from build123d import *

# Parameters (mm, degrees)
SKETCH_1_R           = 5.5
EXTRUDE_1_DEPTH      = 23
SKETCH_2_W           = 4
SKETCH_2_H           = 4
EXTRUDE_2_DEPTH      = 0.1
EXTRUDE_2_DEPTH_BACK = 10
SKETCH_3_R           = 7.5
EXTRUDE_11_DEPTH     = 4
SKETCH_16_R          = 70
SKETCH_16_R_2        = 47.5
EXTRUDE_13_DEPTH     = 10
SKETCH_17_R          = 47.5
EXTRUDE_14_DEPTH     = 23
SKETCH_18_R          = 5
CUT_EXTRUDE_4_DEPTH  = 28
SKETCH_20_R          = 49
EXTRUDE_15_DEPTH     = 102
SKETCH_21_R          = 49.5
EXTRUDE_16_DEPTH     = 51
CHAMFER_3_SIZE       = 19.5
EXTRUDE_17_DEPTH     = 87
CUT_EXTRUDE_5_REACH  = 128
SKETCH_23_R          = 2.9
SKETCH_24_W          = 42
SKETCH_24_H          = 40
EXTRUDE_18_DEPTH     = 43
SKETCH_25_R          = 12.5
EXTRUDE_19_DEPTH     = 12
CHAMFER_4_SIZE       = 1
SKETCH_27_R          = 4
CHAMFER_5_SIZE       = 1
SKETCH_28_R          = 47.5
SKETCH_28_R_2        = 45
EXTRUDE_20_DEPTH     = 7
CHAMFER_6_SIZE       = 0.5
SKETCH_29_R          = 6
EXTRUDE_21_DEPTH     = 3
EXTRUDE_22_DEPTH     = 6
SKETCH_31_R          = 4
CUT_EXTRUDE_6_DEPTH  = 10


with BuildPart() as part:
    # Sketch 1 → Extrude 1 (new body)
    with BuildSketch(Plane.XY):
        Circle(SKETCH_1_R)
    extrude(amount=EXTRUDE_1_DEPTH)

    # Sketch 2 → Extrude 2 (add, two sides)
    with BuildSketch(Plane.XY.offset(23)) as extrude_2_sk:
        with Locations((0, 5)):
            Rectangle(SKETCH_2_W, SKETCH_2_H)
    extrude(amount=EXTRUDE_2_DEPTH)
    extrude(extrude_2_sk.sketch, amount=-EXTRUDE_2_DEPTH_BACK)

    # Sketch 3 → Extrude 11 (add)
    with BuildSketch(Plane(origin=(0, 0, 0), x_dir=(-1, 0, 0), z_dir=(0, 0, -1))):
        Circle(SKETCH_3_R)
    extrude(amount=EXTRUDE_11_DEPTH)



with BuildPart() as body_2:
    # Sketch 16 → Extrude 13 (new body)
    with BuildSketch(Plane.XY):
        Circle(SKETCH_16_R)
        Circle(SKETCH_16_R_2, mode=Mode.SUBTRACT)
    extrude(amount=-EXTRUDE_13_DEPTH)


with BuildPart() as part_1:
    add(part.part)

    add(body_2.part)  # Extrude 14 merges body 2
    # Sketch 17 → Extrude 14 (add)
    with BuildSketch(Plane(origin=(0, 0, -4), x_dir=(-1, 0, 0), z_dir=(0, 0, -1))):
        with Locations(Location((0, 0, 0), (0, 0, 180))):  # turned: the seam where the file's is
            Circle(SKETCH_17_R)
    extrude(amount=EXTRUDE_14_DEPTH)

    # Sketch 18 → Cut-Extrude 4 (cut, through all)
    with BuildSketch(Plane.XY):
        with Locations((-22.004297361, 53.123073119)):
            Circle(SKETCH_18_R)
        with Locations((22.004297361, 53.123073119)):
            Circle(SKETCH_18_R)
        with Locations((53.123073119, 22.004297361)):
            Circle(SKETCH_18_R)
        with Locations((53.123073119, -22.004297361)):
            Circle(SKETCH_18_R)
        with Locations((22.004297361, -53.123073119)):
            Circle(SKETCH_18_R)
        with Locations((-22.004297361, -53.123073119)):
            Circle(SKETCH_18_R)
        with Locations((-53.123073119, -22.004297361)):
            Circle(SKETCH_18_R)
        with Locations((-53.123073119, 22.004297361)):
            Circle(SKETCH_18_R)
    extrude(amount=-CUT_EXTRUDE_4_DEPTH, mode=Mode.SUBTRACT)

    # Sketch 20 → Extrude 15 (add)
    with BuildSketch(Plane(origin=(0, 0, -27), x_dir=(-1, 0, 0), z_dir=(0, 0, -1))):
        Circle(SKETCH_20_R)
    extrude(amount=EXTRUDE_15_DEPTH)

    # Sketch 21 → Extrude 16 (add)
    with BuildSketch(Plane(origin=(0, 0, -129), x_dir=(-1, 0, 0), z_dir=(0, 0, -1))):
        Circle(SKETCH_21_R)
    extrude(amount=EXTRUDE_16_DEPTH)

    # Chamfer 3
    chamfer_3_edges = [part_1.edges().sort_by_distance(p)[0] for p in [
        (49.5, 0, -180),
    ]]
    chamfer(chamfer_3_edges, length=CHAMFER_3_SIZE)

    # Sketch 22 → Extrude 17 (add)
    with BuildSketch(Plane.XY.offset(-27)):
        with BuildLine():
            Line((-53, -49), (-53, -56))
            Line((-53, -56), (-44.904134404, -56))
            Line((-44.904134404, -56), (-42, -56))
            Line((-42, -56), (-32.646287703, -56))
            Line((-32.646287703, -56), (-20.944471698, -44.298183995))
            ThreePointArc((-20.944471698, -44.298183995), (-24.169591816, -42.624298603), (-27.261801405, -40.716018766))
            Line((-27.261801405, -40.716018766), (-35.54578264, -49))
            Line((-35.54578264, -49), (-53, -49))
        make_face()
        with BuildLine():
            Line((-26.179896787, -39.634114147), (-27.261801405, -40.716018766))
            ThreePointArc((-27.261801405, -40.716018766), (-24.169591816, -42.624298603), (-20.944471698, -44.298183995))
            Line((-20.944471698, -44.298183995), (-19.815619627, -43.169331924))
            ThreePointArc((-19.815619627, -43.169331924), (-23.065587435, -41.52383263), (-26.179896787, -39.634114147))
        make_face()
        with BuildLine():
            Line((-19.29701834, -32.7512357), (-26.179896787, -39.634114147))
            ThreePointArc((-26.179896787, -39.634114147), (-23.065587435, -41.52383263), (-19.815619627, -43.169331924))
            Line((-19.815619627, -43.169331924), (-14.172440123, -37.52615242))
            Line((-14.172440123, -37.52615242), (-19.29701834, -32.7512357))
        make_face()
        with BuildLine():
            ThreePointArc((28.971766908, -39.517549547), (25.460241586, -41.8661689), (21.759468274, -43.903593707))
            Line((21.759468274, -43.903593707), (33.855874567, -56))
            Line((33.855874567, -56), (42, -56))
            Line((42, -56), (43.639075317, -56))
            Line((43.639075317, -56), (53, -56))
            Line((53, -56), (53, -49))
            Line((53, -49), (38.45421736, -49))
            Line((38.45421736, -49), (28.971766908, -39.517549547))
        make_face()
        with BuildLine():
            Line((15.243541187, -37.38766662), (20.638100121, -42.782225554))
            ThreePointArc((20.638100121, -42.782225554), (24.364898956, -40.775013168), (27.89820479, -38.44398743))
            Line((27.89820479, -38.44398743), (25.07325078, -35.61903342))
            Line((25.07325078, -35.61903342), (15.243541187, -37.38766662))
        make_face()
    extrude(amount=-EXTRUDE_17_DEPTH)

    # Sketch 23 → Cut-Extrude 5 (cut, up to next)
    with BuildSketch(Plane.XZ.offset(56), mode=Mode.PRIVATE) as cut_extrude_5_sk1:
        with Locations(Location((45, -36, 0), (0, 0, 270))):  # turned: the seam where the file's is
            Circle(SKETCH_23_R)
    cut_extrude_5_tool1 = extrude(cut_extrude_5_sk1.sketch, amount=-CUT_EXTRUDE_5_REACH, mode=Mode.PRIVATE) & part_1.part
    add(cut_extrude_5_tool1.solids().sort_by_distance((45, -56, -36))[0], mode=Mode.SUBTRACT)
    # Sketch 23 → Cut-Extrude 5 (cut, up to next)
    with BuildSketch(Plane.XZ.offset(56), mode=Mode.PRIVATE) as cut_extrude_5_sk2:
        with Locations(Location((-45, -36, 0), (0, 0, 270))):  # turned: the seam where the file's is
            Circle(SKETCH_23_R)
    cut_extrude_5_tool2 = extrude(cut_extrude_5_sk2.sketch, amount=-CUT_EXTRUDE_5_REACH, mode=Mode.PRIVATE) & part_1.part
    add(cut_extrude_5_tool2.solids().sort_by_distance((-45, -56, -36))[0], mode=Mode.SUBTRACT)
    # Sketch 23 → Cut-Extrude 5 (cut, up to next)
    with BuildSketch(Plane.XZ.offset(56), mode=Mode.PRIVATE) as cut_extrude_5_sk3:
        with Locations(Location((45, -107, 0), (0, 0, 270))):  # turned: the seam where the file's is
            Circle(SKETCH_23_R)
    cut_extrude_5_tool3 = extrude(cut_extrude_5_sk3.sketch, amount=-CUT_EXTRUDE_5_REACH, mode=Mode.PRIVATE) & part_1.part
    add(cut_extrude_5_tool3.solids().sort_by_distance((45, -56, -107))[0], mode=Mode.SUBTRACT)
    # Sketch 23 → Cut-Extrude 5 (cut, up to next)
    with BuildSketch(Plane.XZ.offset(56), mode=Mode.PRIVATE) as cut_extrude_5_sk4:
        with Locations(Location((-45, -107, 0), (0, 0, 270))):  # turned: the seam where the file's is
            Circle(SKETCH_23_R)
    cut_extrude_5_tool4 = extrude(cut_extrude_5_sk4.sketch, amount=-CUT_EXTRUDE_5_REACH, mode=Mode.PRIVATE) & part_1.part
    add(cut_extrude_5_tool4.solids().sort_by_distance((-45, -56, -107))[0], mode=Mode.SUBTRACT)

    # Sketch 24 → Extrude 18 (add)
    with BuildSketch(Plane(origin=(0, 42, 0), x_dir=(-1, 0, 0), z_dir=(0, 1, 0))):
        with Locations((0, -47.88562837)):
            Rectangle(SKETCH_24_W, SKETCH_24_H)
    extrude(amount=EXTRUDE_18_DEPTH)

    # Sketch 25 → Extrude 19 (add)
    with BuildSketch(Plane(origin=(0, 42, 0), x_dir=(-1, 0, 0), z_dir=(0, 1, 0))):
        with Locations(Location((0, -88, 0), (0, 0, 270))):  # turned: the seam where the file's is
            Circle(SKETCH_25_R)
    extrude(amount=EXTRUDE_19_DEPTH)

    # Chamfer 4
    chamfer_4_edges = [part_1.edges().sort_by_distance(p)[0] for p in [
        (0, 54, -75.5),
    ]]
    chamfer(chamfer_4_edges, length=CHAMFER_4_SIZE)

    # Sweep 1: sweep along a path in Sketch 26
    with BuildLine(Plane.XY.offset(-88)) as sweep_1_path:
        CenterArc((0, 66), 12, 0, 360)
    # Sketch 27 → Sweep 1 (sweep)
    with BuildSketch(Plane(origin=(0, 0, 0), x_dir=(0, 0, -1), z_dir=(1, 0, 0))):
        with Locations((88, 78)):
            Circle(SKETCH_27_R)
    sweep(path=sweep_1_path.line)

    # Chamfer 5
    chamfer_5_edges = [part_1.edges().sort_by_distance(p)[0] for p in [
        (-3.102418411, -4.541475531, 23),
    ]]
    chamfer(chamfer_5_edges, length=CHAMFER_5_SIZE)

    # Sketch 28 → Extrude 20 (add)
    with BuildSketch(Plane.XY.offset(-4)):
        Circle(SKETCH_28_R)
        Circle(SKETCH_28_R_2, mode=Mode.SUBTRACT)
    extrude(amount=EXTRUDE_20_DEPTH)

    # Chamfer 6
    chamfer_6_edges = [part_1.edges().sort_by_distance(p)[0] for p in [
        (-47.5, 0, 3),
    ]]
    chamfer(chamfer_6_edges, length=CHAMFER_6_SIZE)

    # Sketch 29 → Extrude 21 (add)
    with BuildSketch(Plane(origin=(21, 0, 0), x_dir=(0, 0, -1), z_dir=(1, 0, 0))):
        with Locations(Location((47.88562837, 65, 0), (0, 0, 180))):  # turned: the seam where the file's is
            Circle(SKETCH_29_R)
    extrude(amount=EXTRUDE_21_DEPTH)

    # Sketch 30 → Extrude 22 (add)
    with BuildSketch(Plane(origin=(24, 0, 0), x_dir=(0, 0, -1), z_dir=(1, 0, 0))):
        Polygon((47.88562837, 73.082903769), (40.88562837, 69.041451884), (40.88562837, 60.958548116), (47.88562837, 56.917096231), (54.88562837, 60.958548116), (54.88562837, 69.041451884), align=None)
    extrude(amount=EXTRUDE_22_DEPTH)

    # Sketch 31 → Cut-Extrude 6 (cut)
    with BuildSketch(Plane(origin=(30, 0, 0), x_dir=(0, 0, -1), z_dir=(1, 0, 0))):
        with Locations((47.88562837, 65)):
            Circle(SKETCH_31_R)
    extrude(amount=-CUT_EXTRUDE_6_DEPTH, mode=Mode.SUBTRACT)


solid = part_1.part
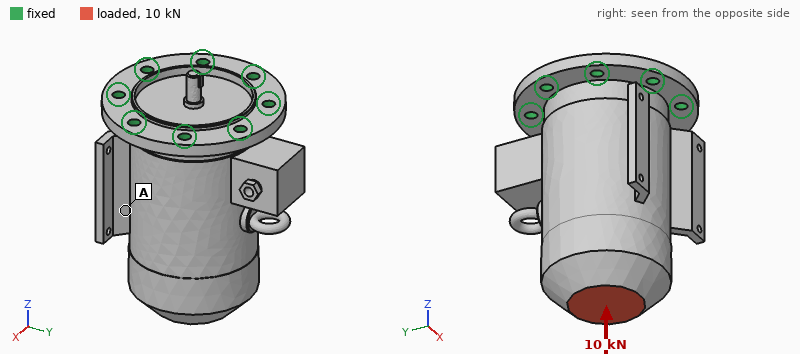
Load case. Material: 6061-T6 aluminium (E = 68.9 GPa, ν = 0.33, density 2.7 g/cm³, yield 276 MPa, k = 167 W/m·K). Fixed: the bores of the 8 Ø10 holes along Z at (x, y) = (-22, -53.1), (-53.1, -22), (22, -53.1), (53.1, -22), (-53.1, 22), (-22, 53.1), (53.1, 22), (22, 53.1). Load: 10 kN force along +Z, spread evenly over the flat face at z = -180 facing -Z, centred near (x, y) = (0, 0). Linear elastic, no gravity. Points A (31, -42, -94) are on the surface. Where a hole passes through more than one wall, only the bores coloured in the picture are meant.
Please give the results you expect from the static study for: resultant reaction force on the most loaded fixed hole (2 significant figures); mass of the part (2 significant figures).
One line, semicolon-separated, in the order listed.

1.5 kN; 4.0 kg
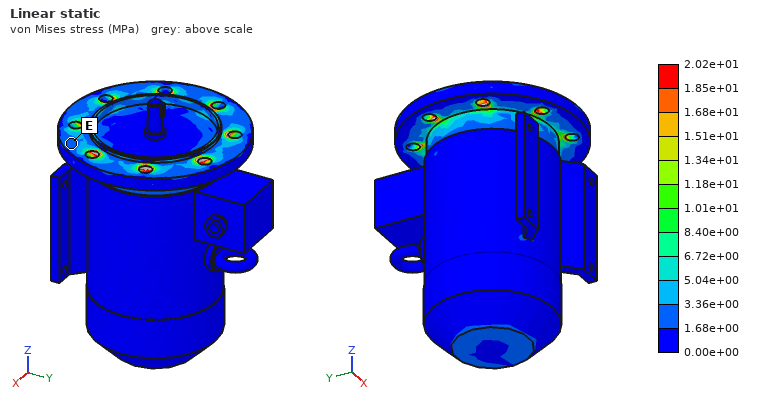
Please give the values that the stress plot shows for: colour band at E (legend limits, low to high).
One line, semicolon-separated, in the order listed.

1.68e+00 to 3.36e+00 MPa
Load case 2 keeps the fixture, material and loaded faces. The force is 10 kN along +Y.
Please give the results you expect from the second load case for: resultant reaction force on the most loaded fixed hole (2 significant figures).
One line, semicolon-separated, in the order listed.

8.6 kN
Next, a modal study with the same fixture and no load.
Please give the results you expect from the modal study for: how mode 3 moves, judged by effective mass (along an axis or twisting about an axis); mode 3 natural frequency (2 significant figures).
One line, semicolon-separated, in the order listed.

along Z; 3700 Hz
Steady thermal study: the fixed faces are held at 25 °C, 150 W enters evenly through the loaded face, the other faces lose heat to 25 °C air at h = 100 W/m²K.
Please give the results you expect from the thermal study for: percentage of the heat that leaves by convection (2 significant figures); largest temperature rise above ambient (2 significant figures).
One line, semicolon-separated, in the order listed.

48 %; 22 K
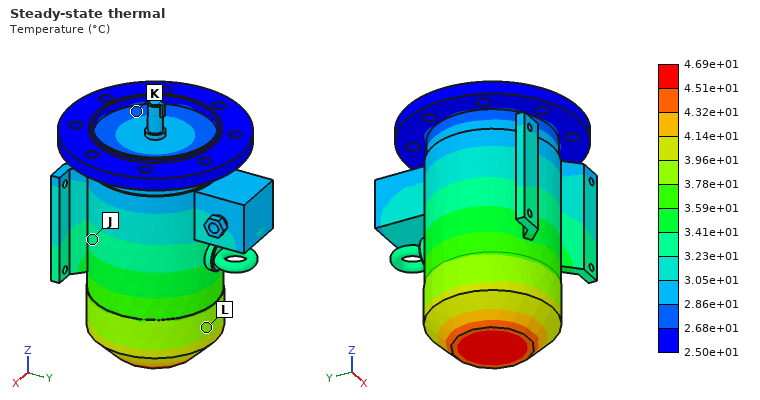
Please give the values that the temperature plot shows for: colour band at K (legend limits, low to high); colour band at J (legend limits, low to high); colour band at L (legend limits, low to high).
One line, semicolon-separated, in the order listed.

2.68e+01 to 2.86e+01 °C; 3.23e+01 to 3.41e+01 °C; 3.78e+01 to 3.96e+01 °C
